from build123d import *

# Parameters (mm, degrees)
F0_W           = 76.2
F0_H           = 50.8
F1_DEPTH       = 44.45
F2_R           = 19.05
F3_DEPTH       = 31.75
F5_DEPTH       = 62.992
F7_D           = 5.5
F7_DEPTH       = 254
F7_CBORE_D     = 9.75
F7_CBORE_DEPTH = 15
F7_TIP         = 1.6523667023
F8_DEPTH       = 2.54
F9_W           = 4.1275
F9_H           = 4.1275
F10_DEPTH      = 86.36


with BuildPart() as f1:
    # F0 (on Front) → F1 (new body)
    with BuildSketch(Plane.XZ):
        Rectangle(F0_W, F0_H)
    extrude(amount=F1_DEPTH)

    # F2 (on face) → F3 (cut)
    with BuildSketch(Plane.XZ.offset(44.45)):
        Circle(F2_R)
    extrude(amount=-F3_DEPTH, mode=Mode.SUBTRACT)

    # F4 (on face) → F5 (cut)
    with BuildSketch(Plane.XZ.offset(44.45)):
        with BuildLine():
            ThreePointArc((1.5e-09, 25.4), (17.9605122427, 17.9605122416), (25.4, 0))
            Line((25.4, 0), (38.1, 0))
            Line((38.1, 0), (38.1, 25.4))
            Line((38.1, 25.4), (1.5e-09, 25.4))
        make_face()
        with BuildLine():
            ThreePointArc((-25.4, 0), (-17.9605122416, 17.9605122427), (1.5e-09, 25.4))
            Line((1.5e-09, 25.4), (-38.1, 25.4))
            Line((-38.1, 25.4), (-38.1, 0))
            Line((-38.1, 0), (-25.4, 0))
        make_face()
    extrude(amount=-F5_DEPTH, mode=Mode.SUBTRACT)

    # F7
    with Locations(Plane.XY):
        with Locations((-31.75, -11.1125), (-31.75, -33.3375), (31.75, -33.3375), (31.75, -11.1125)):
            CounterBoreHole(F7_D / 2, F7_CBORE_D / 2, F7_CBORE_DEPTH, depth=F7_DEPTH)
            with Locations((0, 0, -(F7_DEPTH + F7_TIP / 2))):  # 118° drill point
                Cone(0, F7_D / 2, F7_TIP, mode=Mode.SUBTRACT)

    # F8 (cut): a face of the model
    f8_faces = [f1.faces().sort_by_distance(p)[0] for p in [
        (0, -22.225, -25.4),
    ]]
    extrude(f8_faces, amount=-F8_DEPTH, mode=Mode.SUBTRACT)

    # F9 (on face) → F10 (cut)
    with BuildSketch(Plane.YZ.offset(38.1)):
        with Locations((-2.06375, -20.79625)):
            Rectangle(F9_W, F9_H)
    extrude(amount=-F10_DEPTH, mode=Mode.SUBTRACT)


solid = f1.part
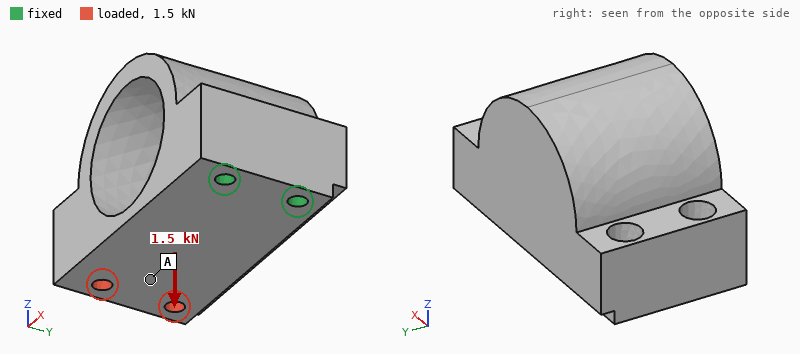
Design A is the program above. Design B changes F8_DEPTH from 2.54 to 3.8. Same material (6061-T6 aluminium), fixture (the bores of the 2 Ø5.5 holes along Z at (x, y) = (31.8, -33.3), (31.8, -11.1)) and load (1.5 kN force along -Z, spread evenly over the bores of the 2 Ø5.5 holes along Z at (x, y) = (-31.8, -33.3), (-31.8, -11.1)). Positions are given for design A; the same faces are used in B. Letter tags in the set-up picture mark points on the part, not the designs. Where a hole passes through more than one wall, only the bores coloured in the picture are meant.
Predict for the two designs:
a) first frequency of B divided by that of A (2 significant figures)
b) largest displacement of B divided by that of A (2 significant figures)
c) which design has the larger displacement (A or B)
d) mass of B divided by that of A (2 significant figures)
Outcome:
0.90
1.3
B
0.95
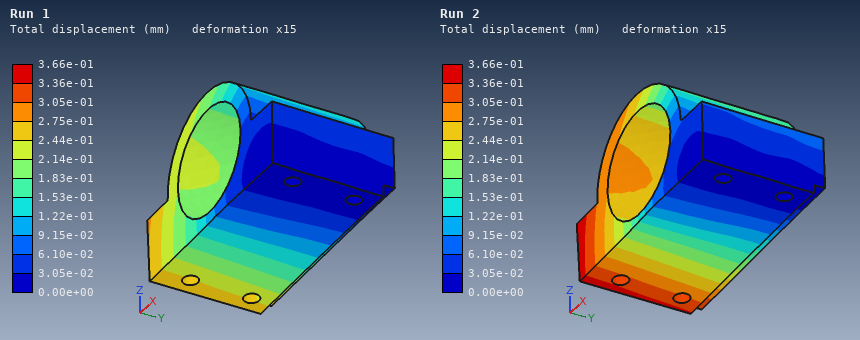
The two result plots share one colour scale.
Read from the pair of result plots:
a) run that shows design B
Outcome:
Run 2
